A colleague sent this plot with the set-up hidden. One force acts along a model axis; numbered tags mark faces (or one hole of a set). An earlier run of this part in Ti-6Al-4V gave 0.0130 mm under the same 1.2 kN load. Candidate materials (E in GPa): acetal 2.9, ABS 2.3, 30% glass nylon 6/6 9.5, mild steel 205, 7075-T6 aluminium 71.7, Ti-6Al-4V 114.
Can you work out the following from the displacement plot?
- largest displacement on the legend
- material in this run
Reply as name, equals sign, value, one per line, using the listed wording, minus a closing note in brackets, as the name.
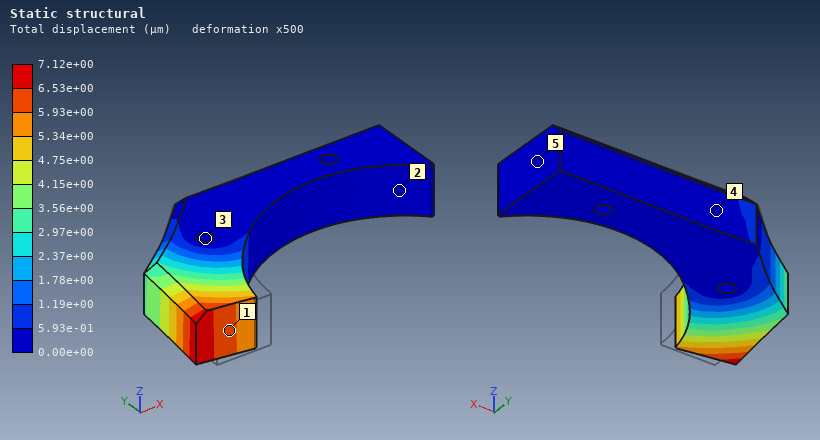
largest displacement on the legend = 7.12e+00 µm
material in this run = mild steel
